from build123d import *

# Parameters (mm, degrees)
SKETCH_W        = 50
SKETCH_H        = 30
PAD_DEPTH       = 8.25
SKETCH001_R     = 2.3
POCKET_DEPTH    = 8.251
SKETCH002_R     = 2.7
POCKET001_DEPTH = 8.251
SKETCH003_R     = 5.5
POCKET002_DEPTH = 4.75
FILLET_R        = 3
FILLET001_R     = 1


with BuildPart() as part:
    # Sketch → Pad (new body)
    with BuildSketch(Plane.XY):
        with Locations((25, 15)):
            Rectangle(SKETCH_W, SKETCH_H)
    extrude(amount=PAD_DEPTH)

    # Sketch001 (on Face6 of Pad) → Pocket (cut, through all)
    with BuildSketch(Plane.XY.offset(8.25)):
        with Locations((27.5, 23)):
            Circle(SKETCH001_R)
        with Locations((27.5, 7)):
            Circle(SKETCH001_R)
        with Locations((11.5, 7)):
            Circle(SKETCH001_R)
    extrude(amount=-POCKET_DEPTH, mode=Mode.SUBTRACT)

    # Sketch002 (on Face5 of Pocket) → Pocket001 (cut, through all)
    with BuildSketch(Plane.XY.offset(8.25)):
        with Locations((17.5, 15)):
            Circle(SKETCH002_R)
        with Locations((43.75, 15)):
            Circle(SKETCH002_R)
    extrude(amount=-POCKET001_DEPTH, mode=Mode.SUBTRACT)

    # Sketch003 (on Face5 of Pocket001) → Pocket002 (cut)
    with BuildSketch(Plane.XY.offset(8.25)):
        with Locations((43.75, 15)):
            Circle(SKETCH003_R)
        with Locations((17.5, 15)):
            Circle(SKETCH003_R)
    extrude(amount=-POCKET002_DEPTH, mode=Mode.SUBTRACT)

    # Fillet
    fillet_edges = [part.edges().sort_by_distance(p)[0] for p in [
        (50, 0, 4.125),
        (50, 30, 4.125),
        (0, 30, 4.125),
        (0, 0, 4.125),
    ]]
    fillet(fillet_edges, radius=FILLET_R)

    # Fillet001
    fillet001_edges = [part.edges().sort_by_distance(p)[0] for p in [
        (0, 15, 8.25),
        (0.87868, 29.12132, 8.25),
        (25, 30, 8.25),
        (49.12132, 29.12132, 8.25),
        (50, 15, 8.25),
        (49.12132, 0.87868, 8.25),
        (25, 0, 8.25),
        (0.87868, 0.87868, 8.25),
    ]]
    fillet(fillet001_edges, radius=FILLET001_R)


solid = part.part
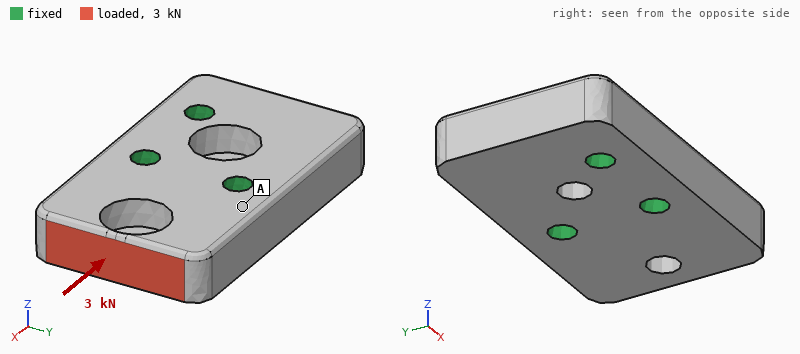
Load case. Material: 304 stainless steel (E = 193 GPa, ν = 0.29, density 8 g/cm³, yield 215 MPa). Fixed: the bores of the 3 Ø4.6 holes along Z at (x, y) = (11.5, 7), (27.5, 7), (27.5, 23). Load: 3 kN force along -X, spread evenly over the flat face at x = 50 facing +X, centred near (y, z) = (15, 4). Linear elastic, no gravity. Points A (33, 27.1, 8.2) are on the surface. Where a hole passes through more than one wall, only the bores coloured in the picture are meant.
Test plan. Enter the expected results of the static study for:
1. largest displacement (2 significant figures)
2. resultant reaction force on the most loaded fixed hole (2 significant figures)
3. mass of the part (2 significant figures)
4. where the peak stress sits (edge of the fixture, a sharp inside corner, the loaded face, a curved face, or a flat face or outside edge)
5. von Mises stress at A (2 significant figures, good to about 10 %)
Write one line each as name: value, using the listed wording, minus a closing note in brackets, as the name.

largest displacement: 7.2 µm
resultant reaction force on the most loaded fixed hole: 1.5 kN
mass of the part: 86 g
where the peak stress sits: the loaded face
von Mises stress at A: 9.4 MPa
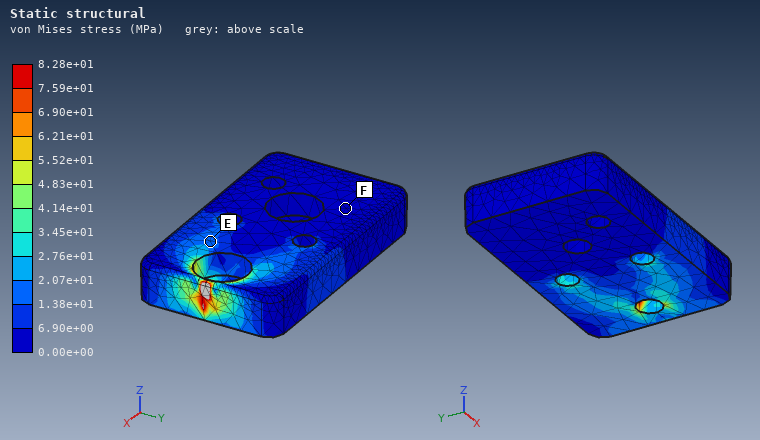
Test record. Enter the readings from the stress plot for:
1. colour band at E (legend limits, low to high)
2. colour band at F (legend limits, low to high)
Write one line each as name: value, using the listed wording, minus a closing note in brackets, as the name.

colour band at E: 1.38e+01 to 2.07e+01 MPa
colour band at F: 0.00e+00 to 6.90e+00 MPa
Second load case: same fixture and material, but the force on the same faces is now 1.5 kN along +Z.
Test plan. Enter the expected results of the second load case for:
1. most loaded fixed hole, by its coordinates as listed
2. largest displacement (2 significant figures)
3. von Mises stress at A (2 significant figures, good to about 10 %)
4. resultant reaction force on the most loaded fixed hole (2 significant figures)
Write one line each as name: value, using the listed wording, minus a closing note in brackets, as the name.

most loaded fixed hole, by its coordinates as listed: (27.5, 7)
largest displacement: 29 µm
von Mises stress at A: 75 MPa
resultant reaction force on the most loaded fixed hole: 900 N
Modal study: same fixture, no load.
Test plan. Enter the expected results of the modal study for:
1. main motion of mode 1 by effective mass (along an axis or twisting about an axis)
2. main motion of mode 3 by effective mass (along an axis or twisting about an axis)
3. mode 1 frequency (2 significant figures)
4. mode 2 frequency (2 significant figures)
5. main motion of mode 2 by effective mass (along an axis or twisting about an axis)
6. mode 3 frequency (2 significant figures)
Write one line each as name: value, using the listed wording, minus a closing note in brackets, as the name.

main motion of mode 1 by effective mass: along Z
main motion of mode 3 by effective mass: twisting about X
mode 1 frequency: 13 kHz
mode 2 frequency: 16 kHz
main motion of mode 2 by effective mass: along Z
mode 3 frequency: 19 kHz
